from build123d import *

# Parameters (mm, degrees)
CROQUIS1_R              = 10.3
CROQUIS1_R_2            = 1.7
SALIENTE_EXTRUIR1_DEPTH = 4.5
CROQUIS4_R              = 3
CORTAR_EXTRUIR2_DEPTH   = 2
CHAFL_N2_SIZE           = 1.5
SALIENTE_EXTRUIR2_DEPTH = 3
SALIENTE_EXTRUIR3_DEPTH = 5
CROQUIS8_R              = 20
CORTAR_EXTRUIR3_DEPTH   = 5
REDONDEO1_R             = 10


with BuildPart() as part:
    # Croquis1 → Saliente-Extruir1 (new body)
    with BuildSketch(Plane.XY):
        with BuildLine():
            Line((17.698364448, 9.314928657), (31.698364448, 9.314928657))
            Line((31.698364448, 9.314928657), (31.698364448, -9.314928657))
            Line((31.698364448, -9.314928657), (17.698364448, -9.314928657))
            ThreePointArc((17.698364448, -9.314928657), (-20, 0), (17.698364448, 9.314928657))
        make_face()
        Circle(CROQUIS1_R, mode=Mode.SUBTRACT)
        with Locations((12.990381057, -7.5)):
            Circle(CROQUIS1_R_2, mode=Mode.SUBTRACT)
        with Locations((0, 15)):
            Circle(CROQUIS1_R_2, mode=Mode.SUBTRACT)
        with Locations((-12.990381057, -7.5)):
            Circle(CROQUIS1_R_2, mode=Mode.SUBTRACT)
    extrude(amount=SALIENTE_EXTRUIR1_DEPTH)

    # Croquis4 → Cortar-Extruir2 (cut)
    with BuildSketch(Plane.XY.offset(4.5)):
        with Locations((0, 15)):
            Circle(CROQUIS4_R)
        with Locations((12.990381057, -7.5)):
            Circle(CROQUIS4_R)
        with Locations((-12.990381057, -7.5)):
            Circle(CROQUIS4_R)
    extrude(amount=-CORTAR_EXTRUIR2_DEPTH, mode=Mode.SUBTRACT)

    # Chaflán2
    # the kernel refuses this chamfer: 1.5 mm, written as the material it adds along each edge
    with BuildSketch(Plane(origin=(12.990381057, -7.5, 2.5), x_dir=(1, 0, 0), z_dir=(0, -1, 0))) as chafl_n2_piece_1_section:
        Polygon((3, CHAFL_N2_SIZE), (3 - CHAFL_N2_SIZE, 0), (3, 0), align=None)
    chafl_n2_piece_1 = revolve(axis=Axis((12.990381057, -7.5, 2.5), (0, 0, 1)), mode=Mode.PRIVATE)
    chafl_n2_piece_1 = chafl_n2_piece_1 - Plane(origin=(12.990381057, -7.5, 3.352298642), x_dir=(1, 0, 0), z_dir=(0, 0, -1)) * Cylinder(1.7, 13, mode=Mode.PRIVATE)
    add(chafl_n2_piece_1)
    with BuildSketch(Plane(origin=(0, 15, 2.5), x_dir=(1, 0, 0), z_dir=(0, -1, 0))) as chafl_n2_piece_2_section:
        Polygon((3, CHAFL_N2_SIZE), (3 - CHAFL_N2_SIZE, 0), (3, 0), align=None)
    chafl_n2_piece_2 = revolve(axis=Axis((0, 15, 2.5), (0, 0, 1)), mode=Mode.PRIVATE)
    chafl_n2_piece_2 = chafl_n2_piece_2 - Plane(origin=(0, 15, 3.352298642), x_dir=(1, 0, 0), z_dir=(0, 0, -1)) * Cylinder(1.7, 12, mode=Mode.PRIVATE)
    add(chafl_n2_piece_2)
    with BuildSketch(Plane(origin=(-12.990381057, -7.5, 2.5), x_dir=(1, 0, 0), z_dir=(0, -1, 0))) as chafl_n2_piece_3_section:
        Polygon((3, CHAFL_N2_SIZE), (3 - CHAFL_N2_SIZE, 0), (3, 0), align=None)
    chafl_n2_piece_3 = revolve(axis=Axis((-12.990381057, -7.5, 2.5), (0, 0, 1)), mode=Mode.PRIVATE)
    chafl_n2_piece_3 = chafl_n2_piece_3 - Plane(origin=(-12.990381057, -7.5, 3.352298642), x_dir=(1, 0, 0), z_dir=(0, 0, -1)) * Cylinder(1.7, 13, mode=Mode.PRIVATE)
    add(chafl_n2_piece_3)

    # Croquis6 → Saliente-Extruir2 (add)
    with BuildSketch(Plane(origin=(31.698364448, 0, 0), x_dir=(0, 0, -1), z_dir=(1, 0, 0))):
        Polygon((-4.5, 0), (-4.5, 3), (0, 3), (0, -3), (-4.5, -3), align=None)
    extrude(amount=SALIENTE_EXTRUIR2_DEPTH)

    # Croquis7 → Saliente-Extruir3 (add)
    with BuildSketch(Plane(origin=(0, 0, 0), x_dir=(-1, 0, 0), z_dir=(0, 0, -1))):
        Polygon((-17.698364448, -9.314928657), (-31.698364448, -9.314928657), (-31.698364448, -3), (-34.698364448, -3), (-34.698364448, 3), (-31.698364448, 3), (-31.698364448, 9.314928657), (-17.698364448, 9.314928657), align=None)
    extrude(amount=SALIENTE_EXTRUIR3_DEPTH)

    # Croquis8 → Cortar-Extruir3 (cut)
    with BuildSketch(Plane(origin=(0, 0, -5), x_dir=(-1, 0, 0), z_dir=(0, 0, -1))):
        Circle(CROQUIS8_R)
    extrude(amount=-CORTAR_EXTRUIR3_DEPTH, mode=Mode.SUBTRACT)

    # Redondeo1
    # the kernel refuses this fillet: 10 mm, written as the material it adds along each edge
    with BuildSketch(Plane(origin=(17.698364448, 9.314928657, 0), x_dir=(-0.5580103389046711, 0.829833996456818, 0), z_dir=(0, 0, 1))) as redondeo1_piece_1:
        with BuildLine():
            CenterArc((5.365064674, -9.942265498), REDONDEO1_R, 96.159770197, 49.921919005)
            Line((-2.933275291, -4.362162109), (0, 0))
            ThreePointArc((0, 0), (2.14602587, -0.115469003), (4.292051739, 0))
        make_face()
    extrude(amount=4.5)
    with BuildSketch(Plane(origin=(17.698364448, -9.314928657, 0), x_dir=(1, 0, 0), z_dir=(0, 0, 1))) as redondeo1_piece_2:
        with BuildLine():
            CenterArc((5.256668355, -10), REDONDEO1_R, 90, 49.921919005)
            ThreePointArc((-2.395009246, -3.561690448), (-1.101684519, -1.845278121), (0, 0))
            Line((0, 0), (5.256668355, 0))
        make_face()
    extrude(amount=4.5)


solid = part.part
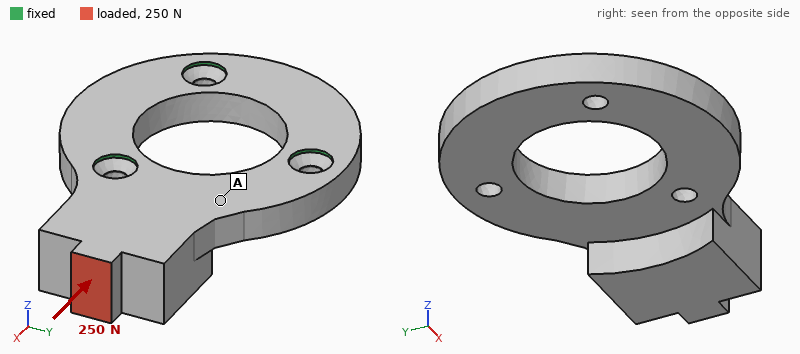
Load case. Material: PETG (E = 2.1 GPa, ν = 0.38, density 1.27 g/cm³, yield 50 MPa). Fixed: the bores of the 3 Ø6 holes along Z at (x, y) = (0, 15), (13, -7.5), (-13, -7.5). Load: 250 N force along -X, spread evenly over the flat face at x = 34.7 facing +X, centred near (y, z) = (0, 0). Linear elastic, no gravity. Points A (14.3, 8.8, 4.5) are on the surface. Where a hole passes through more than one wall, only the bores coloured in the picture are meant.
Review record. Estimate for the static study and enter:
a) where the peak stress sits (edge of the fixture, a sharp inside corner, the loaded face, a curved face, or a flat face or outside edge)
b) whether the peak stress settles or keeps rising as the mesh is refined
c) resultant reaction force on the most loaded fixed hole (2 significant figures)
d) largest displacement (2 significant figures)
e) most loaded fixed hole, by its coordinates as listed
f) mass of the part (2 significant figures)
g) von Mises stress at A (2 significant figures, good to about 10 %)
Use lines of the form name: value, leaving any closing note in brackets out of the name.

where the peak stress sits: edge of the fixture
whether the peak stress settles or keeps rising as the mesh is refined: keeps rising
resultant reaction force on the most loaded fixed hole: 130 N
largest displacement: 0.58 mm
most loaded fixed hole, by its coordinates as listed: (13, -7.5)
mass of the part: 8.1 g
von Mises stress at A: 3.4 MPa
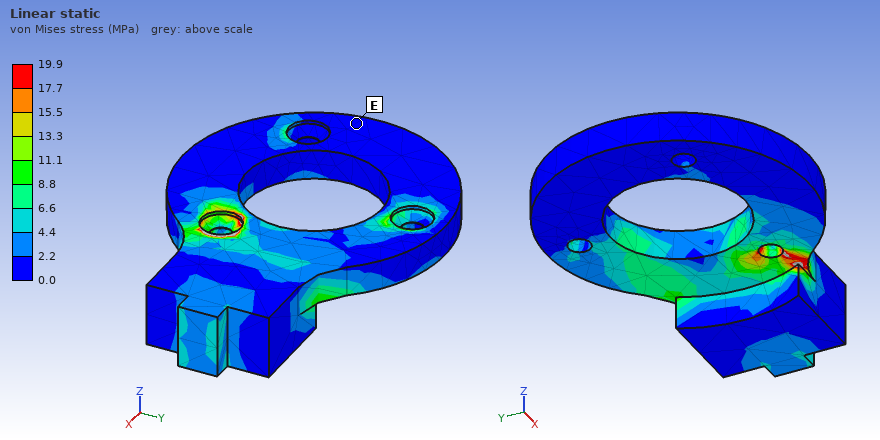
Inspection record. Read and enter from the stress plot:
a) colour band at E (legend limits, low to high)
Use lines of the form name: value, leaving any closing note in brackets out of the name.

colour band at E: 0.0 to 2.2 MPa
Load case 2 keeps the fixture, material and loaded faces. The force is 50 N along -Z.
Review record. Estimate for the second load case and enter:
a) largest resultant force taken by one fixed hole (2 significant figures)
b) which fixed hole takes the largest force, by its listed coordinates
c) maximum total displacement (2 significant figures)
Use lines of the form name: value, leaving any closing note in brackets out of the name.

largest resultant force taken by one fixed hole: 70 N
which fixed hole takes the largest force, by its listed coordinates: (13, -7.5)
maximum total displacement: 0.79 mm
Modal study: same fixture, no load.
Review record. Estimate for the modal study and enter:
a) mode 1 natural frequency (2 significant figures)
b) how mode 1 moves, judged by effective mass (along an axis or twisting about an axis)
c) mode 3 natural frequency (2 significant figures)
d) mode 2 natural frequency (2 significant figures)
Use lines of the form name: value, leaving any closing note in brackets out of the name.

mode 1 natural frequency: 1200 Hz
how mode 1 moves, judged by effective mass: along Z
mode 3 natural frequency: 3900 Hz
mode 2 natural frequency: 3400 Hz
